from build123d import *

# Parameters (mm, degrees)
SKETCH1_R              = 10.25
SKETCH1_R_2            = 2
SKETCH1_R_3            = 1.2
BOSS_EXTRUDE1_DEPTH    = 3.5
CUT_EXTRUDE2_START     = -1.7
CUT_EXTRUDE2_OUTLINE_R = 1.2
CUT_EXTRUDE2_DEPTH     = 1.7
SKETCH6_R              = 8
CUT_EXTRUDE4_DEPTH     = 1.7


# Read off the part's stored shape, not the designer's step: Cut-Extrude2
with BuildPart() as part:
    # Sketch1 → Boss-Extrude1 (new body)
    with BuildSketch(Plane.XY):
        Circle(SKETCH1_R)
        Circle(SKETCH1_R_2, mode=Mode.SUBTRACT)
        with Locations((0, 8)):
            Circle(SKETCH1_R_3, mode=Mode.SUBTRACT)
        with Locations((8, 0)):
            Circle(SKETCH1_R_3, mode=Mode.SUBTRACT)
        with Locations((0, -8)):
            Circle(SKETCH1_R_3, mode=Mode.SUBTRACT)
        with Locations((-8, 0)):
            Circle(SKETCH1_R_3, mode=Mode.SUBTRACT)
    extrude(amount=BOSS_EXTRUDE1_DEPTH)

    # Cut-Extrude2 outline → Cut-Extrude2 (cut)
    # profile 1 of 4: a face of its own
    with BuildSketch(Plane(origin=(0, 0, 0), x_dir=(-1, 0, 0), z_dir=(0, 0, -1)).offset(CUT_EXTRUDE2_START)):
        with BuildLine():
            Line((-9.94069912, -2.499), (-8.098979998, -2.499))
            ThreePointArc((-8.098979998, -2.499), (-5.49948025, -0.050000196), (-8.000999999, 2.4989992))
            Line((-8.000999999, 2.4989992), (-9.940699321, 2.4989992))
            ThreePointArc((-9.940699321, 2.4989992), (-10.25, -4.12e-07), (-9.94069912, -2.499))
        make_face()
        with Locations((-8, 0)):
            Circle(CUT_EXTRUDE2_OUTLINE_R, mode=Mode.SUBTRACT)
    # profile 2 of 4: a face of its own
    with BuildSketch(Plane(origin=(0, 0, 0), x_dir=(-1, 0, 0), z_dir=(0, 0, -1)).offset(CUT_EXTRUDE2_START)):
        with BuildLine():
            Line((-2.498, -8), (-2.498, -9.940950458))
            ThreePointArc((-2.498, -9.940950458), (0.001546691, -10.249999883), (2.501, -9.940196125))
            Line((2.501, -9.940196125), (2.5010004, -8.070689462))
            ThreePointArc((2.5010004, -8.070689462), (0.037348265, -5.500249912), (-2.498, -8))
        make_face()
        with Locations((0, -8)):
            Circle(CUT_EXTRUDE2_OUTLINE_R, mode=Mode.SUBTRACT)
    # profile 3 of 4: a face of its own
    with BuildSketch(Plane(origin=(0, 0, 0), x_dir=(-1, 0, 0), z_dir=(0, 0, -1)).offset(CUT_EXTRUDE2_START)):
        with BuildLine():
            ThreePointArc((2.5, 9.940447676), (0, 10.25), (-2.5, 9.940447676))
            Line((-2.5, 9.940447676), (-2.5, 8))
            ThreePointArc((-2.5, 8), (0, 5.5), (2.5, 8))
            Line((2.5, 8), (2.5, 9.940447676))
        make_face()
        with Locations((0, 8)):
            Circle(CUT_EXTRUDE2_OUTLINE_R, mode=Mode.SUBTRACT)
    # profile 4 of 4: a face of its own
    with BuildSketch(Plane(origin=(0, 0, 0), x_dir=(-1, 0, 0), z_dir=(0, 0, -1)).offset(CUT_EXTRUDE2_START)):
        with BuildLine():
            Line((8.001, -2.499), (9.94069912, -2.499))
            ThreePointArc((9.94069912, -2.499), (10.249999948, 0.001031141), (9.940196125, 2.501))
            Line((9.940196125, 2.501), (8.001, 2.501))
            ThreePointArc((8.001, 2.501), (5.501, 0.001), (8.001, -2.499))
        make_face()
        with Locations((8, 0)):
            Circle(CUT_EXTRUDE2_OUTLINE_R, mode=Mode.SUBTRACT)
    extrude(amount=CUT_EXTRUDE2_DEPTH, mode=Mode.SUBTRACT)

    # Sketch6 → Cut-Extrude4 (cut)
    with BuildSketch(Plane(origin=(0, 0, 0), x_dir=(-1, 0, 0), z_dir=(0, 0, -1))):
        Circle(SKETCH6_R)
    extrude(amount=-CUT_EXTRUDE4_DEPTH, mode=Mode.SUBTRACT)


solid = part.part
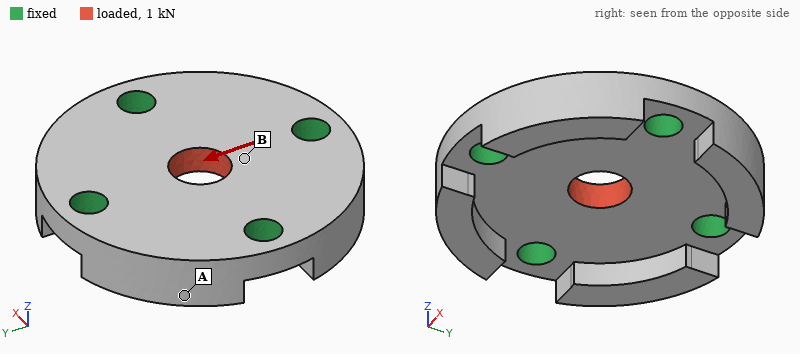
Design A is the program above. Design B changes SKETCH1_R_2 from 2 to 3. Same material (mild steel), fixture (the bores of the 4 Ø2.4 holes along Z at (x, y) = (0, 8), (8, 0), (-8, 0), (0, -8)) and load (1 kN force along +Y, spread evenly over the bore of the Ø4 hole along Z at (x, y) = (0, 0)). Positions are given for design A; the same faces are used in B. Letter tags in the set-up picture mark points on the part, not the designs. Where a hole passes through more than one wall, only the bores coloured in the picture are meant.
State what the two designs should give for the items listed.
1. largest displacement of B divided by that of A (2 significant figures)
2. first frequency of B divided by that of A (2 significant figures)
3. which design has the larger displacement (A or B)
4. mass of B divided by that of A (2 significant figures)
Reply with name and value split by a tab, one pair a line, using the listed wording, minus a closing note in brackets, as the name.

largest displacement of B divided by that of A	0.80
first frequency of B divided by that of A	1.0
which design has the larger displacement	A
mass of B divided by that of A	0.96
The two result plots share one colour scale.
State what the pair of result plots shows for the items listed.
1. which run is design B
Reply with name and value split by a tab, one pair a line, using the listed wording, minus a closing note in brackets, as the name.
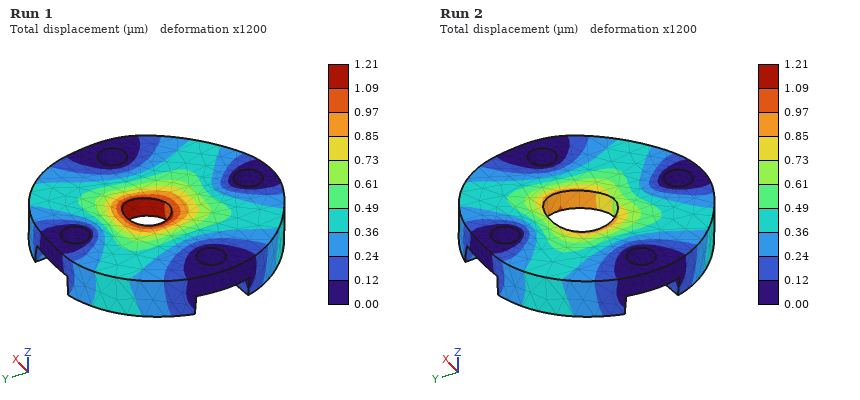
which run is design B	Run 2
